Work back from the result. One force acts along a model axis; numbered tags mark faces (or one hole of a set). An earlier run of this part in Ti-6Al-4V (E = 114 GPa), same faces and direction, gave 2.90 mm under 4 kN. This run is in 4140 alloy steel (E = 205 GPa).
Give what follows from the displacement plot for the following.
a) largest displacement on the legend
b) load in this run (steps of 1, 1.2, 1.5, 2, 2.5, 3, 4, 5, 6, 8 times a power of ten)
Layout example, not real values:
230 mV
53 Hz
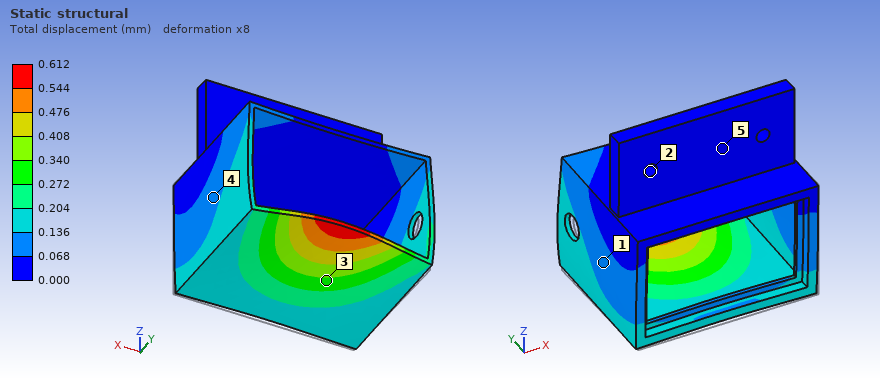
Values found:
0.612 mm
1.5 kN
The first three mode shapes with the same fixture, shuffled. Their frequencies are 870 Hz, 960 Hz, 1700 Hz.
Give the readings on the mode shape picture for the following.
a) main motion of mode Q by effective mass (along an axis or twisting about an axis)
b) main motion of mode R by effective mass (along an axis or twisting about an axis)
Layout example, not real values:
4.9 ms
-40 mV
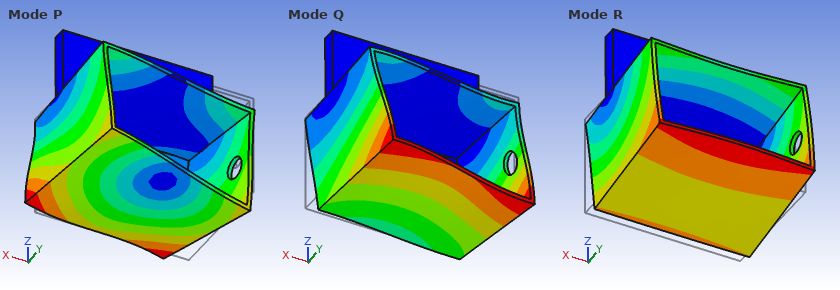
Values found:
along X
along Y
